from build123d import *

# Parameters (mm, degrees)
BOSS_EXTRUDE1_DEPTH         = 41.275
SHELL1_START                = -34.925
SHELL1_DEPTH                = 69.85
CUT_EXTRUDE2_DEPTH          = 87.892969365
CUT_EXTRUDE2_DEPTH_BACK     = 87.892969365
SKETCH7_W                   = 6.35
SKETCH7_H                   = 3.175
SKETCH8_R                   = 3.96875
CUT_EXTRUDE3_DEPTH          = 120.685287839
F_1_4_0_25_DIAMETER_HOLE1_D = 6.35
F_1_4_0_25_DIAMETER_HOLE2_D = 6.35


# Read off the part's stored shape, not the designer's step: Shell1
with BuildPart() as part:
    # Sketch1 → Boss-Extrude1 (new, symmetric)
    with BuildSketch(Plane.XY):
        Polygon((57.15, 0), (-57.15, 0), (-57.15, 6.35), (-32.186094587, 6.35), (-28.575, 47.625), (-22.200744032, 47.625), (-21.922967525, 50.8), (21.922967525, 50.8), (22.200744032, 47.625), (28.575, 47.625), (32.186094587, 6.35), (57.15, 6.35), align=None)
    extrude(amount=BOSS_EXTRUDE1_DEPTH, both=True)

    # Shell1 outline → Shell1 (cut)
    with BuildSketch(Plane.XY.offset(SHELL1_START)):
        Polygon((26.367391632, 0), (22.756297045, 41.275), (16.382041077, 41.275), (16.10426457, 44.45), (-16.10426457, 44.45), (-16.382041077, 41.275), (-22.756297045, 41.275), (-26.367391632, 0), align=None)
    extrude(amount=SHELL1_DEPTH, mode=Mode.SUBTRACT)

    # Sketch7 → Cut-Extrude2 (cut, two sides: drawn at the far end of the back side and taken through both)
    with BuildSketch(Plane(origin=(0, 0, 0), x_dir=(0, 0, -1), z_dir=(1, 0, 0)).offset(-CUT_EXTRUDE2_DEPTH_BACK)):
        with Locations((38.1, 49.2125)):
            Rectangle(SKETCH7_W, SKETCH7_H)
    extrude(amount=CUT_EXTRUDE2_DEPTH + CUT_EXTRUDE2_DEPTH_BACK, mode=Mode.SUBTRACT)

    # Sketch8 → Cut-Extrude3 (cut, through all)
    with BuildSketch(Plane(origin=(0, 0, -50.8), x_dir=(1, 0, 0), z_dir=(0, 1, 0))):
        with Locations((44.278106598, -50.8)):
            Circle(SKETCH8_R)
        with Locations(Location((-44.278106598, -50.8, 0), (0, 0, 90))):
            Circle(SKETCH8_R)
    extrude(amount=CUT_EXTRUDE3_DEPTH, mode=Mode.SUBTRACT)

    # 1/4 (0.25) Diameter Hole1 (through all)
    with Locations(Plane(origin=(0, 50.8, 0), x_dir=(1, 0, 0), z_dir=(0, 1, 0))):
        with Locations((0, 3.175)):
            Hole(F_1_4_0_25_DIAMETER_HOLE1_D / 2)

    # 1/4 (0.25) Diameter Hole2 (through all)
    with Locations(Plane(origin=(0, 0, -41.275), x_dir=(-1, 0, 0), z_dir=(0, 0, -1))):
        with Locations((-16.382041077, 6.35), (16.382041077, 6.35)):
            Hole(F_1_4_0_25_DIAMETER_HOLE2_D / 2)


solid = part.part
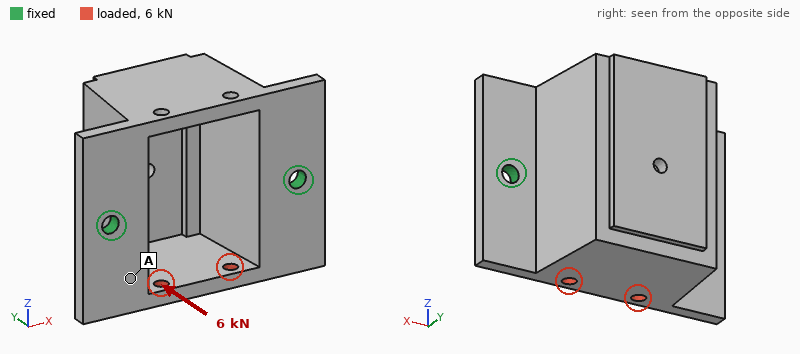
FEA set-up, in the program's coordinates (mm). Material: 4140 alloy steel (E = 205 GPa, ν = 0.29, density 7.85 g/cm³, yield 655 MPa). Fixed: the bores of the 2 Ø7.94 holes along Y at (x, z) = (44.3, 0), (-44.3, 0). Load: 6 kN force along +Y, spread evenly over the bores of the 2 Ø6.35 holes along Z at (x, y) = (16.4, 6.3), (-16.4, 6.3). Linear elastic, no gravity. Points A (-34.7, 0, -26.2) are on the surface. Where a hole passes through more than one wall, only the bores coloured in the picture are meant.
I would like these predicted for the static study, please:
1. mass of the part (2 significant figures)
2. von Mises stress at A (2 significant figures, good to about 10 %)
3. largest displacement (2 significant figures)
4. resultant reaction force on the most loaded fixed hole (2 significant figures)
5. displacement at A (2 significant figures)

1000 g
57 MPa
0.25 mm
3.3 kN
0.11 mm
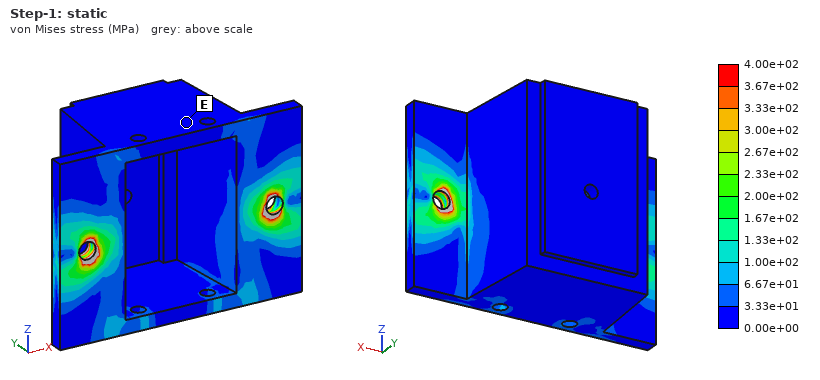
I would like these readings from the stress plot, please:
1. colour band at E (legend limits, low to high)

0.00e+00 to 3.33e+01 MPa
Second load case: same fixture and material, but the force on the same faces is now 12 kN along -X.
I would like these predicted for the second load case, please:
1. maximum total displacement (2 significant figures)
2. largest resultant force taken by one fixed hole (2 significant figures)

92 µm
6.4 kN
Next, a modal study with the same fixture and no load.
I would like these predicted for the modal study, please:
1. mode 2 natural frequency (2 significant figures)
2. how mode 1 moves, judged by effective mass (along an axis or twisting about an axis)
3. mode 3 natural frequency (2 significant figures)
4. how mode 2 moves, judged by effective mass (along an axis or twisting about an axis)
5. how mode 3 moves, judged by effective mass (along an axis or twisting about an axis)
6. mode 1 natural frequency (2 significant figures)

3500 Hz
along Z
3700 Hz
along X
along Y
1000 Hz
